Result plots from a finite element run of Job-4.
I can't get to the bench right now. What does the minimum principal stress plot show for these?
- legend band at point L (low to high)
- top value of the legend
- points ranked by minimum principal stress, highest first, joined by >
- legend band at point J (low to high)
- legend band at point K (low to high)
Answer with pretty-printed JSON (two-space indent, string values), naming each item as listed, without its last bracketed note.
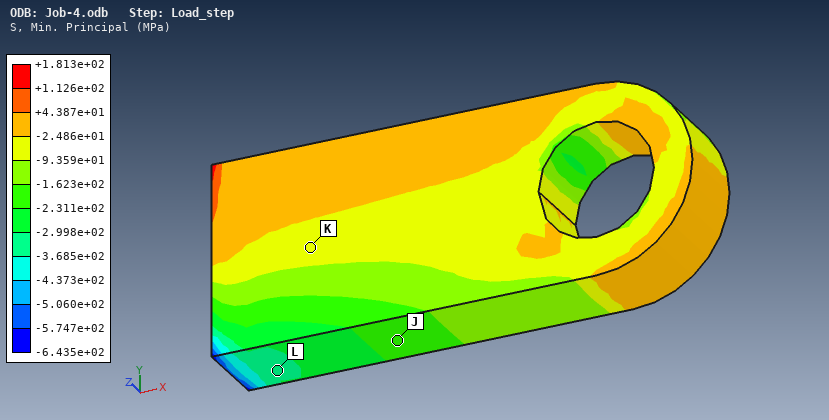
{
  "legend band at point L": "-3.685e+02 to -2.998e+02 MPa",
  "top value of the legend": "+1.813e+02 MPa",
  "points ranked by minimum principal stress, highest first, joined by >": "K > J > L",
  "legend band at point J": "-2.311e+02 to -1.623e+02 MPa",
  "legend band at point K": "-9.359e+01 to -2.486e+01 MPa"
}
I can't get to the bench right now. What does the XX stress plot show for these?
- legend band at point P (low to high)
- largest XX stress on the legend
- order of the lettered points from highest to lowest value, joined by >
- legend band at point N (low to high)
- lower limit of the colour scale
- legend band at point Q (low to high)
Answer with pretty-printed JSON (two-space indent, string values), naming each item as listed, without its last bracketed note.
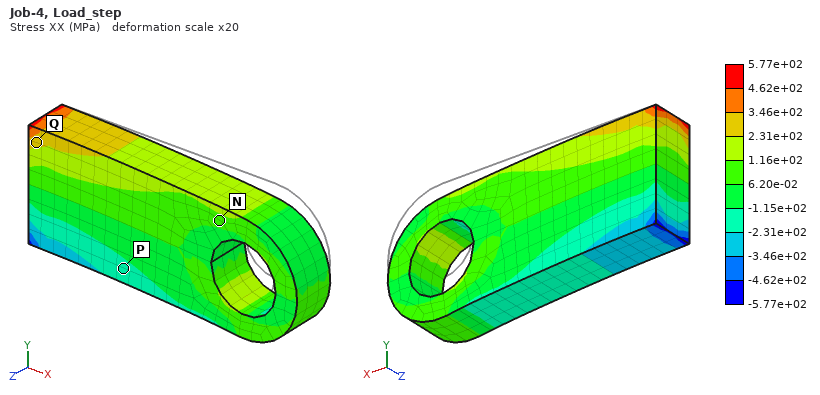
{
  "legend band at point P": "-2.31e+02 to -1.15e+02 MPa",
  "largest XX stress on the legend": "5.77e+02 MPa",
  "order of the lettered points from highest to lowest value, joined by >": "Q > N > P",
  "legend band at point N": "6.20e-02 to 1.16e+02 MPa",
  "lower limit of the colour scale": "-5.77e+02 MPa",
  "legend band at point Q": "2.31e+02 to 3.46e+02 MPa"
}
